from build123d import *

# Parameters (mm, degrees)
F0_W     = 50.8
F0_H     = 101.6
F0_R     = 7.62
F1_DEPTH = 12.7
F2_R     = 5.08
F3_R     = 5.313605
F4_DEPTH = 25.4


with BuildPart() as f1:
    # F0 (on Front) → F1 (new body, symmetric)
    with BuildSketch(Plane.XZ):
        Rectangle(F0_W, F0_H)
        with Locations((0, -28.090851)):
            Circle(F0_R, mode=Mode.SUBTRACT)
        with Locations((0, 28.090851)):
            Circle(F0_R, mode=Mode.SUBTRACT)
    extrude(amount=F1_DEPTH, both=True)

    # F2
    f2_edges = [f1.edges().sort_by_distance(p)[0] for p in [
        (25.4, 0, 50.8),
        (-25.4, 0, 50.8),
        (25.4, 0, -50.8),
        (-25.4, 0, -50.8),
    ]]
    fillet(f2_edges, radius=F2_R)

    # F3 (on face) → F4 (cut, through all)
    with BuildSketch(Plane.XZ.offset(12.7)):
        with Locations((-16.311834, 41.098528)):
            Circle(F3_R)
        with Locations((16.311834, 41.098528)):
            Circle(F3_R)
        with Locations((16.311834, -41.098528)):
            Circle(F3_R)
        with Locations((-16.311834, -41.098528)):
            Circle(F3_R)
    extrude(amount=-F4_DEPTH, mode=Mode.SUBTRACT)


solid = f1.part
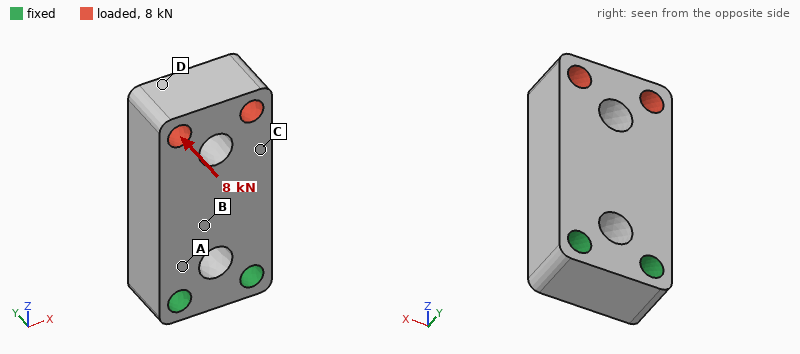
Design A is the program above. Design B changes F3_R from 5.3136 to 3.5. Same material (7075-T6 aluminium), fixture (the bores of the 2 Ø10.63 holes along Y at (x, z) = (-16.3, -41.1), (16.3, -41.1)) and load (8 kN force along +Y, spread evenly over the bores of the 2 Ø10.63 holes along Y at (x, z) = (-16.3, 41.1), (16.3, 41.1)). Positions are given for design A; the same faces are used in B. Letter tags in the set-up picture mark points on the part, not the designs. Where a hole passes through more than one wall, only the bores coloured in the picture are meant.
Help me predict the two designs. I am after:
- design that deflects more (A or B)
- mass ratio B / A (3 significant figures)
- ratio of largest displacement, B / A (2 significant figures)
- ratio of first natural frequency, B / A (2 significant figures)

B
1.05
1.1
0.91
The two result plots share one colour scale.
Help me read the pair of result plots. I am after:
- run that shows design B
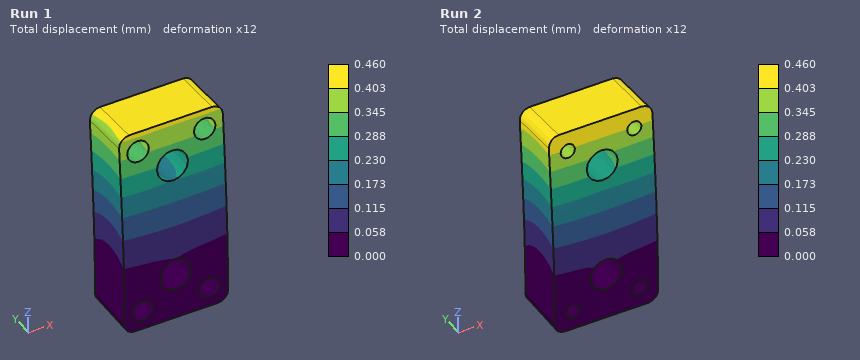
Run 2
